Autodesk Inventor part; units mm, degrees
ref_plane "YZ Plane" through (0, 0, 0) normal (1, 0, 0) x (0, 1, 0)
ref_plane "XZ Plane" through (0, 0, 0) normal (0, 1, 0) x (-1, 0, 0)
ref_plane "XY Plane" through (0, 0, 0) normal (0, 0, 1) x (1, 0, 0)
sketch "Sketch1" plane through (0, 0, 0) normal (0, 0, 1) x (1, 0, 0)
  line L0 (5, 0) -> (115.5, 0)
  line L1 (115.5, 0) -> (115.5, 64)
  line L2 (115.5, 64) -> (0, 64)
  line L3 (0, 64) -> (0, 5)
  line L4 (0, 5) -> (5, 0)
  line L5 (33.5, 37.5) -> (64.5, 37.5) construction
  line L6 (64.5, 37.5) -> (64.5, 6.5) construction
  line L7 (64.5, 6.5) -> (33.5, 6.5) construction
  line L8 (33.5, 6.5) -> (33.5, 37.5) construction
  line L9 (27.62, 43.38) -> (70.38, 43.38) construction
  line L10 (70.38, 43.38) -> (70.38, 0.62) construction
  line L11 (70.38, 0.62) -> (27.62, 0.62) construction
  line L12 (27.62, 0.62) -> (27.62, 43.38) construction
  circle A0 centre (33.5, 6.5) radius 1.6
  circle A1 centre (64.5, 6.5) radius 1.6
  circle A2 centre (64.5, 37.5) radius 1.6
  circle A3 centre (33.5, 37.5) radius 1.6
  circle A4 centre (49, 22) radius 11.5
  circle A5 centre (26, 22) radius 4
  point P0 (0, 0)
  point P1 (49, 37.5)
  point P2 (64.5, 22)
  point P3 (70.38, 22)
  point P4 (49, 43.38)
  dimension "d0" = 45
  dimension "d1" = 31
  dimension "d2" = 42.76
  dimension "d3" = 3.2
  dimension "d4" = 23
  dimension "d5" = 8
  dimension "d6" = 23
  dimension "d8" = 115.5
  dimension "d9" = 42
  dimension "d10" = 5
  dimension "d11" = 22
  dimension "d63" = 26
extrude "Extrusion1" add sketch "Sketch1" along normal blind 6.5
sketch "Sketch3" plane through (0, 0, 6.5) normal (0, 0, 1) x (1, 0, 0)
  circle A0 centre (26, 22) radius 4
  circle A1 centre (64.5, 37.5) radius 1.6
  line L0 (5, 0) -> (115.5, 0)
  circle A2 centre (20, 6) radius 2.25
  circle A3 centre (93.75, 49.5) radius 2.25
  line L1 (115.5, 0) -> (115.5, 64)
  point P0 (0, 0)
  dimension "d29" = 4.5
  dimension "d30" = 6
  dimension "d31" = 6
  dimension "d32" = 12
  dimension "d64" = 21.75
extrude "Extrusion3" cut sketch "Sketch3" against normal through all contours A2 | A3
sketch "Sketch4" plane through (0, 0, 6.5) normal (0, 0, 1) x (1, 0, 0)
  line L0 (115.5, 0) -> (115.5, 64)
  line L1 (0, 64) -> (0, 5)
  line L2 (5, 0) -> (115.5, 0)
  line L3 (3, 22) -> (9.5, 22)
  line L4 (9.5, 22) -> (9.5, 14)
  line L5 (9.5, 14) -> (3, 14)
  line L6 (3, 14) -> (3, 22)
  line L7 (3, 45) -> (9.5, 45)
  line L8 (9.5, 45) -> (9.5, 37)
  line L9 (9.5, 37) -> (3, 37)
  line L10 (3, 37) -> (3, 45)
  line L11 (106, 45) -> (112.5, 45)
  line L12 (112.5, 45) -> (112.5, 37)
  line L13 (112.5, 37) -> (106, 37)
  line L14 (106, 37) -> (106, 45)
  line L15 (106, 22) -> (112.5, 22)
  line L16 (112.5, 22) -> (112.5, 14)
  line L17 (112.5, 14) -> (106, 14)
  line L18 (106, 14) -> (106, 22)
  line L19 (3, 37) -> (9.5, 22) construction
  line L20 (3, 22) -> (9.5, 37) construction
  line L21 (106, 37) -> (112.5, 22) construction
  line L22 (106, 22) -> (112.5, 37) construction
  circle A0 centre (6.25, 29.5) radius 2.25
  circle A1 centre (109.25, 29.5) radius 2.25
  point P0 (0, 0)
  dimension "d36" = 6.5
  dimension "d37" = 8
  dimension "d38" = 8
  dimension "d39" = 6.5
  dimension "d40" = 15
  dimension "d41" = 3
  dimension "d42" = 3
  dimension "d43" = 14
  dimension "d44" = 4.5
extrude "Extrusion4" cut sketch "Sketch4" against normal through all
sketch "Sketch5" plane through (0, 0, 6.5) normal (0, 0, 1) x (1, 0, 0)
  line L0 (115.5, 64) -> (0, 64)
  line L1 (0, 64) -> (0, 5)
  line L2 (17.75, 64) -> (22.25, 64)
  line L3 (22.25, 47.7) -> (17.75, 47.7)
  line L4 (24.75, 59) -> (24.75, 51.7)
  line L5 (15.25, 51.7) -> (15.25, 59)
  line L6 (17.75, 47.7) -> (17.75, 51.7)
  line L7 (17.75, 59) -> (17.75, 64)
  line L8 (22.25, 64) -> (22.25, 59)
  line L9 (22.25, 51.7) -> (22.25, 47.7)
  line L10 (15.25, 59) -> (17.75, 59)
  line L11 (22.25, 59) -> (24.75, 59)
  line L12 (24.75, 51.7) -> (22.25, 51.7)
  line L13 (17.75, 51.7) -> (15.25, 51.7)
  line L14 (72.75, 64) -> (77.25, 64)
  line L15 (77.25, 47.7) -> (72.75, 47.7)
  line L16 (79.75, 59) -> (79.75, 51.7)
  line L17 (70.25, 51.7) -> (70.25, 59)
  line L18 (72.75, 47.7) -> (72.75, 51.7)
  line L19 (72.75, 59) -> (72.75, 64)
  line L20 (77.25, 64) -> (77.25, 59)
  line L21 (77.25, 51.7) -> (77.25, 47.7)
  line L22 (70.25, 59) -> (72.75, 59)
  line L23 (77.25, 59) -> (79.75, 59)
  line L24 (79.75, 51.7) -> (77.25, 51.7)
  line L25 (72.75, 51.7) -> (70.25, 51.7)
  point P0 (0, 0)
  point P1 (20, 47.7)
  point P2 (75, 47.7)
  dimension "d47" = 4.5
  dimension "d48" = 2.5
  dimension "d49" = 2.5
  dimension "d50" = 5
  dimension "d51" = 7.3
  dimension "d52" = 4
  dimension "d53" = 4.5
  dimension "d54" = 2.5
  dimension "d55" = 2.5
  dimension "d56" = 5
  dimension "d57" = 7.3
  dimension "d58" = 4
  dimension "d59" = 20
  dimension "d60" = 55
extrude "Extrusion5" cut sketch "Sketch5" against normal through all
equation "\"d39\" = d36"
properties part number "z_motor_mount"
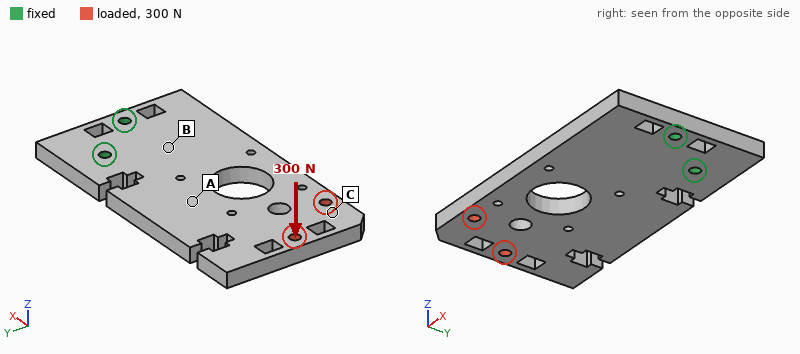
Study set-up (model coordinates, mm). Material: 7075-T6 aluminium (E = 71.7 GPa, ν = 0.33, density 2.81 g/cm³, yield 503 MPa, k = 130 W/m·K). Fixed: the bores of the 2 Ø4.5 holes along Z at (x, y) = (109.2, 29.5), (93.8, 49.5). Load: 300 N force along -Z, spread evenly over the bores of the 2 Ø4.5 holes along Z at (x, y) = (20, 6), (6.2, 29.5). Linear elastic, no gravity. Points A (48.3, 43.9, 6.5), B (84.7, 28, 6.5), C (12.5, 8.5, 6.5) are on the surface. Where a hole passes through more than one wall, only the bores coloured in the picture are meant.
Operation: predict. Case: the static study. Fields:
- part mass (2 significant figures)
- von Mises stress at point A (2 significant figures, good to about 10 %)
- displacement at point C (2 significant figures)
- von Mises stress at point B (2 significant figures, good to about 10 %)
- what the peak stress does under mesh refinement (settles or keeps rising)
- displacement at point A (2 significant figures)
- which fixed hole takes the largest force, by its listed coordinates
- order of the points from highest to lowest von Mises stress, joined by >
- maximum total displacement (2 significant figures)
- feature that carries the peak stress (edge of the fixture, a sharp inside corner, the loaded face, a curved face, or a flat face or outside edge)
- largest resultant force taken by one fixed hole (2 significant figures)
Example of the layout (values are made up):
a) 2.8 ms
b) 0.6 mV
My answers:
a) 120 g
b) 35 MPa
c) 1.0 mm
d) 54 MPa
e) keeps rising
f) 0.35 mm
g) (93.8, 49.5)
h) B > A > C
i) 1.3 mm
j) edge of the fixture
k) 460 N
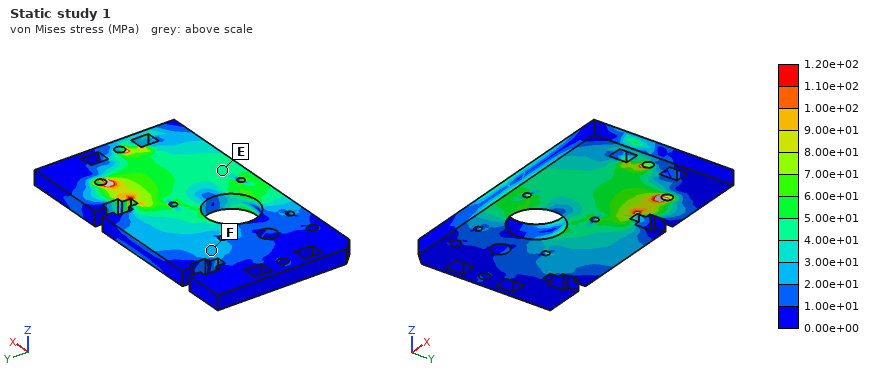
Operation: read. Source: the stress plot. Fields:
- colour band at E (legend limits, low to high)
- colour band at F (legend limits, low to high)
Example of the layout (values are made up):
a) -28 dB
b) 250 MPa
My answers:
a) 4.00e+01 to 5.00e+01 MPa
b) 2.00e+01 to 3.00e+01 MPa
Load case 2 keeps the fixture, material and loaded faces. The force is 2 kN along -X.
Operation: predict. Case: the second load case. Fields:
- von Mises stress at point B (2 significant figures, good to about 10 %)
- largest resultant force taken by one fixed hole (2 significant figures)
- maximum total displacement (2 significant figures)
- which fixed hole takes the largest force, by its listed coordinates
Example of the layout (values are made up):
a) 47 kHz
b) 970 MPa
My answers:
a) 11 MPa
b) 2.4 kN
c) 57 µm
d) (109.2, 29.5)
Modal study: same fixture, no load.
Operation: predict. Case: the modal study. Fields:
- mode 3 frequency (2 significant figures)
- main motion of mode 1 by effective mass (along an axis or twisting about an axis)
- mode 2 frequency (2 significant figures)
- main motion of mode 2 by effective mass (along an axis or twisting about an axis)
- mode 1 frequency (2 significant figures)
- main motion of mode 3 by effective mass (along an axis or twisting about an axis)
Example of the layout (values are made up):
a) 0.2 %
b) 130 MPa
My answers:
a) 2400 Hz
b) along Z
c) 1400 Hz
d) twisting about X
e) 490 Hz
f) along Y
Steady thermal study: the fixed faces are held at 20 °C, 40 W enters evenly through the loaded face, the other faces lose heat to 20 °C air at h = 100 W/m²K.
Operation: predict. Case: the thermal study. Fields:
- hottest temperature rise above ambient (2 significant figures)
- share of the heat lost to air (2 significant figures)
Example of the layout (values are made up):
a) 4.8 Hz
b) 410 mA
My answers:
a) 49 K
b) 75 %
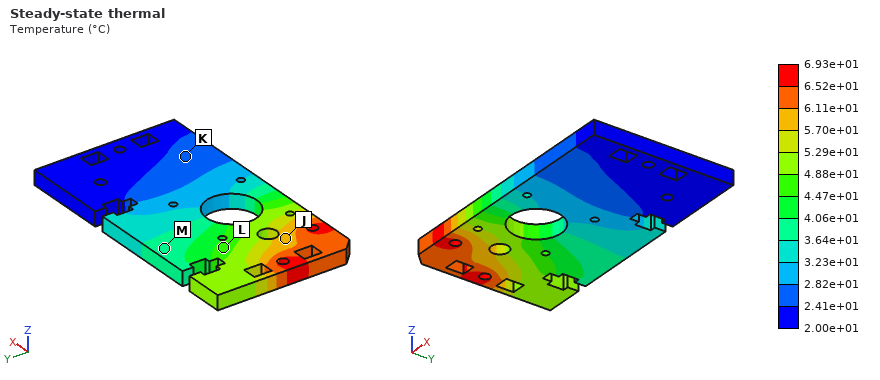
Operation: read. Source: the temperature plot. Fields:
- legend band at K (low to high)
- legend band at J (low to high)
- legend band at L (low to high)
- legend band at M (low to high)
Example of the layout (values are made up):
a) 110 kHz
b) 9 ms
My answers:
a) 2.41e+01 to 2.82e+01 °C
b) 5.70e+01 to 6.11e+01 °C
c) 4.47e+01 to 4.88e+01 °C
d) 3.64e+01 to 4.06e+01 °C
